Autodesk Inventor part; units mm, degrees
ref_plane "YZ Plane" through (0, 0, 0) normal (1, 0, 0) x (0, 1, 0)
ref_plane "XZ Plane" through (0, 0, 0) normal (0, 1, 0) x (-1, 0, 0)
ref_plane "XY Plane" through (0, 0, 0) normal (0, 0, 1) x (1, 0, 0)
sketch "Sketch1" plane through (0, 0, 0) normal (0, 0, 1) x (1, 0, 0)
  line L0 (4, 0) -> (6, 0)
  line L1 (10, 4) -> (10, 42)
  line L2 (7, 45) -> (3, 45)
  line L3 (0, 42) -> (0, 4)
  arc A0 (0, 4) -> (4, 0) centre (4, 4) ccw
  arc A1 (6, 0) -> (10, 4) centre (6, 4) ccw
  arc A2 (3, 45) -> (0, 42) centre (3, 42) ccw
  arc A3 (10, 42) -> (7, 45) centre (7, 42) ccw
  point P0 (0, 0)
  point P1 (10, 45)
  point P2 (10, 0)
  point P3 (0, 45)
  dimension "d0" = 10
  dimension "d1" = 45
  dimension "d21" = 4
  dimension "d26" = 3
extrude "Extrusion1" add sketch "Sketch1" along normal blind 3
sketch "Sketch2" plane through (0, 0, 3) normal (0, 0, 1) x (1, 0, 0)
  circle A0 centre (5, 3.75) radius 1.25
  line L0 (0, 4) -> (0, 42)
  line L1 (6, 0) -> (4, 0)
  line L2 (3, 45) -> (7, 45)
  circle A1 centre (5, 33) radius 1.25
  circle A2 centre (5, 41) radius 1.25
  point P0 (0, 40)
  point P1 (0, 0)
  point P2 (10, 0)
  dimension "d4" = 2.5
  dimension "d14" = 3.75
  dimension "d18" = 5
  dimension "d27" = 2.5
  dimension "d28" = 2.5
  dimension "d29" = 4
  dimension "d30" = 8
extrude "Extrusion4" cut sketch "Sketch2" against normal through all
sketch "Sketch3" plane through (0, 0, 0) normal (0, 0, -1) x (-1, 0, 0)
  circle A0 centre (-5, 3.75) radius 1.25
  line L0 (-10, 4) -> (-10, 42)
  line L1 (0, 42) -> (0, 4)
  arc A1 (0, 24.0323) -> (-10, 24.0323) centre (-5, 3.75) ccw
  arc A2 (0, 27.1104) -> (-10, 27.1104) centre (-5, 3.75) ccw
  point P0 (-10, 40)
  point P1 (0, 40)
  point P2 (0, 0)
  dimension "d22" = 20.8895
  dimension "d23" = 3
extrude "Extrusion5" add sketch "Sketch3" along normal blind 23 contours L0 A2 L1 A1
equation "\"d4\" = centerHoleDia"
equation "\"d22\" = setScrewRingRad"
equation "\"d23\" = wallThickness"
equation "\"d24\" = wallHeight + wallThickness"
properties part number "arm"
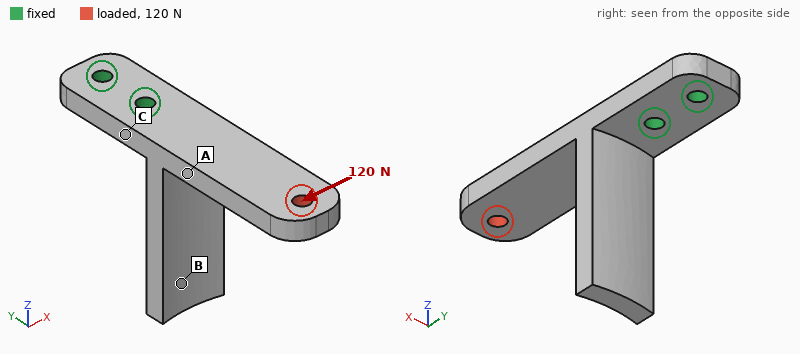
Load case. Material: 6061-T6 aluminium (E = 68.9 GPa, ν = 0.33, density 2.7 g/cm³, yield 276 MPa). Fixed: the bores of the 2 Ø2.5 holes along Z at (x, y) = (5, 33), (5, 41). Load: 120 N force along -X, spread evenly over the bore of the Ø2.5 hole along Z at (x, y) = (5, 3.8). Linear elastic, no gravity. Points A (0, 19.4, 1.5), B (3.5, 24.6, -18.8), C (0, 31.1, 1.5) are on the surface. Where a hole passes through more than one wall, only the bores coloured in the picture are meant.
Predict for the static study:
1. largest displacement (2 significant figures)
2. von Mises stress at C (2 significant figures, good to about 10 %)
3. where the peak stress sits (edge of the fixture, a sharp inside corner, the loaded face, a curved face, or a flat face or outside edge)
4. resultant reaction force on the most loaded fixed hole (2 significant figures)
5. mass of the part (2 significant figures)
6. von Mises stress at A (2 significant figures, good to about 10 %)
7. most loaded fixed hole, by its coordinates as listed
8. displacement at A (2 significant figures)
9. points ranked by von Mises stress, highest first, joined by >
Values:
98 µm
64 MPa
edge of the fixture
380 N
5.3 g
38 MPa
(5, 33)
32 µm
C > A > B
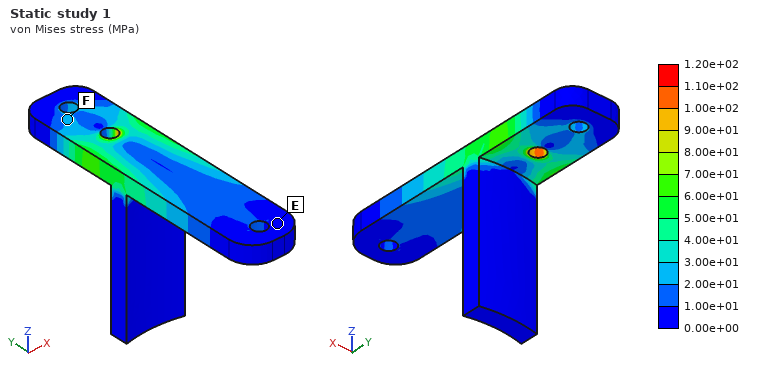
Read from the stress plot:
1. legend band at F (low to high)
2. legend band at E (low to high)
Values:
2.00e+01 to 3.00e+01 MPa
0.00e+00 to 1.00e+01 MPa
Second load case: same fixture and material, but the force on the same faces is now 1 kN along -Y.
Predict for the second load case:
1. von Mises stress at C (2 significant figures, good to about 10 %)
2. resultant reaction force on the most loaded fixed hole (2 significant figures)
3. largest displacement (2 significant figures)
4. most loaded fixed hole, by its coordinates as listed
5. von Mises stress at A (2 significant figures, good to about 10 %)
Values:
18 MPa
840 N
19 µm
(5, 33)
33 MPa
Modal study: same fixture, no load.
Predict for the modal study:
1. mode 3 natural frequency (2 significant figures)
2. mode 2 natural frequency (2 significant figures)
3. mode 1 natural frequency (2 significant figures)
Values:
4400 Hz
4300 Hz
2100 Hz
